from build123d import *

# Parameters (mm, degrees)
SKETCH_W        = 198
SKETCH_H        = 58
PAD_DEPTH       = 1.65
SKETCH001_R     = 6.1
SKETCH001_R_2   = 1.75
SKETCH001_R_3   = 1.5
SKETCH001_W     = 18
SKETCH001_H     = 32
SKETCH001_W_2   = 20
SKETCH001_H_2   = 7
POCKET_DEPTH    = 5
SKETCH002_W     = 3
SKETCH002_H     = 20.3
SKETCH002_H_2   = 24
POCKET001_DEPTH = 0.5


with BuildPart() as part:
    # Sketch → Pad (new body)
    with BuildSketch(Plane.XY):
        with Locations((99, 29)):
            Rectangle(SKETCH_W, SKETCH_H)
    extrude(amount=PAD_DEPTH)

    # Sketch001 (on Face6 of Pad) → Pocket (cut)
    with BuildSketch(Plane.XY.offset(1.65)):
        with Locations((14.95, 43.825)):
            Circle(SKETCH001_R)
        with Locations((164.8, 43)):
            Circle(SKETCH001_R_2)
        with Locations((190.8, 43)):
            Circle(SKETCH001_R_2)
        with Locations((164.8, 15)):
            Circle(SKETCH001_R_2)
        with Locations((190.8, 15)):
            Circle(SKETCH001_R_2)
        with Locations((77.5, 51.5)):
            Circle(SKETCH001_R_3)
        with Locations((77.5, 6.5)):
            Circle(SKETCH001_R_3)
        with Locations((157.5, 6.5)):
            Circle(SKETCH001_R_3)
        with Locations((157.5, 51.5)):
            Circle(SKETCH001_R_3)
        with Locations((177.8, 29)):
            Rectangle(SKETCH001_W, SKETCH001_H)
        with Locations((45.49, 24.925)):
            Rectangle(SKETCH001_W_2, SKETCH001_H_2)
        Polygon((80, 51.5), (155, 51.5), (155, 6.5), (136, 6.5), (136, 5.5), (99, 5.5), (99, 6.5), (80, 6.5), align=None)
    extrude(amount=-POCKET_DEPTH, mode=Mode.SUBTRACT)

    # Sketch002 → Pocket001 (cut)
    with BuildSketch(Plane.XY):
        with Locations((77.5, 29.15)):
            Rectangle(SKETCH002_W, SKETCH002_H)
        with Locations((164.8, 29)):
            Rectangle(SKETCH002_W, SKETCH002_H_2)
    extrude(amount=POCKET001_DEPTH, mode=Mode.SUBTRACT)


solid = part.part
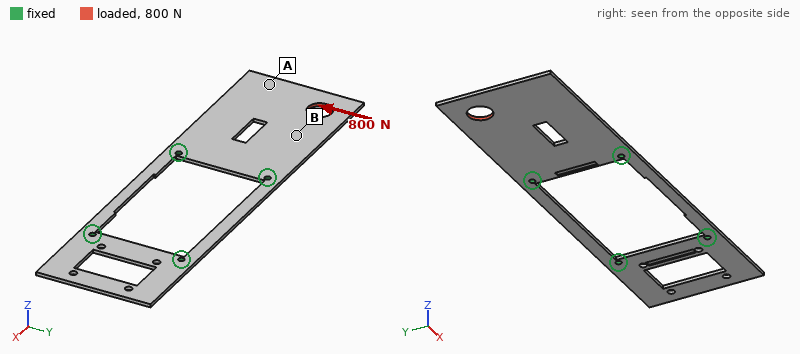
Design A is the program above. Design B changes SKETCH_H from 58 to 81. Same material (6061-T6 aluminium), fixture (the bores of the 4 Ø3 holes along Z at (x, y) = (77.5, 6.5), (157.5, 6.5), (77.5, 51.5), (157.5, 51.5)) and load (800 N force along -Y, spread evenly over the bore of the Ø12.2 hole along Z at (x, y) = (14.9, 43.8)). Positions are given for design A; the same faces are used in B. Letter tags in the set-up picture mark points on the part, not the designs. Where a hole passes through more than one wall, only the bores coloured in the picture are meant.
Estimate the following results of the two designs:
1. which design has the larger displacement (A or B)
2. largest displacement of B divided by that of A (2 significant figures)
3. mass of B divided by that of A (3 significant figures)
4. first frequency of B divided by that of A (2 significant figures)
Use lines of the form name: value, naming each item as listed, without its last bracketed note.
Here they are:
which design has the larger displacement: A
largest displacement of B divided by that of A: 0.69
mass of B divided by that of A: 1.64
first frequency of B divided by that of A: 1.0
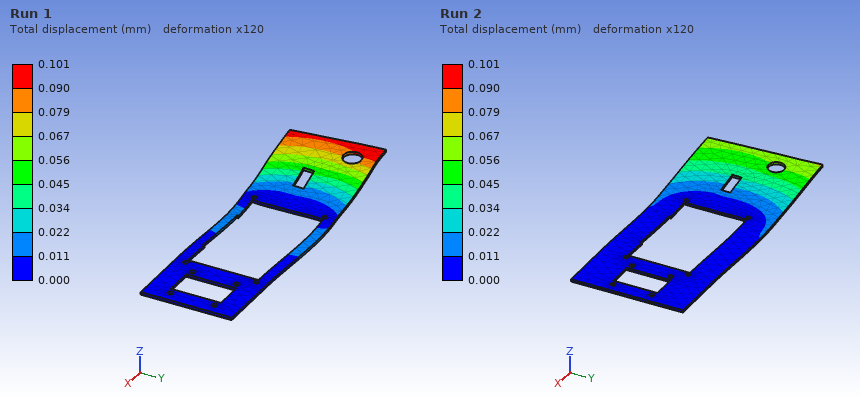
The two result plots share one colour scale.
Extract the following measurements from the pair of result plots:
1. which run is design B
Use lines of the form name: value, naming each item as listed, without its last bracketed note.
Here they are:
which run is design B: Run 2
